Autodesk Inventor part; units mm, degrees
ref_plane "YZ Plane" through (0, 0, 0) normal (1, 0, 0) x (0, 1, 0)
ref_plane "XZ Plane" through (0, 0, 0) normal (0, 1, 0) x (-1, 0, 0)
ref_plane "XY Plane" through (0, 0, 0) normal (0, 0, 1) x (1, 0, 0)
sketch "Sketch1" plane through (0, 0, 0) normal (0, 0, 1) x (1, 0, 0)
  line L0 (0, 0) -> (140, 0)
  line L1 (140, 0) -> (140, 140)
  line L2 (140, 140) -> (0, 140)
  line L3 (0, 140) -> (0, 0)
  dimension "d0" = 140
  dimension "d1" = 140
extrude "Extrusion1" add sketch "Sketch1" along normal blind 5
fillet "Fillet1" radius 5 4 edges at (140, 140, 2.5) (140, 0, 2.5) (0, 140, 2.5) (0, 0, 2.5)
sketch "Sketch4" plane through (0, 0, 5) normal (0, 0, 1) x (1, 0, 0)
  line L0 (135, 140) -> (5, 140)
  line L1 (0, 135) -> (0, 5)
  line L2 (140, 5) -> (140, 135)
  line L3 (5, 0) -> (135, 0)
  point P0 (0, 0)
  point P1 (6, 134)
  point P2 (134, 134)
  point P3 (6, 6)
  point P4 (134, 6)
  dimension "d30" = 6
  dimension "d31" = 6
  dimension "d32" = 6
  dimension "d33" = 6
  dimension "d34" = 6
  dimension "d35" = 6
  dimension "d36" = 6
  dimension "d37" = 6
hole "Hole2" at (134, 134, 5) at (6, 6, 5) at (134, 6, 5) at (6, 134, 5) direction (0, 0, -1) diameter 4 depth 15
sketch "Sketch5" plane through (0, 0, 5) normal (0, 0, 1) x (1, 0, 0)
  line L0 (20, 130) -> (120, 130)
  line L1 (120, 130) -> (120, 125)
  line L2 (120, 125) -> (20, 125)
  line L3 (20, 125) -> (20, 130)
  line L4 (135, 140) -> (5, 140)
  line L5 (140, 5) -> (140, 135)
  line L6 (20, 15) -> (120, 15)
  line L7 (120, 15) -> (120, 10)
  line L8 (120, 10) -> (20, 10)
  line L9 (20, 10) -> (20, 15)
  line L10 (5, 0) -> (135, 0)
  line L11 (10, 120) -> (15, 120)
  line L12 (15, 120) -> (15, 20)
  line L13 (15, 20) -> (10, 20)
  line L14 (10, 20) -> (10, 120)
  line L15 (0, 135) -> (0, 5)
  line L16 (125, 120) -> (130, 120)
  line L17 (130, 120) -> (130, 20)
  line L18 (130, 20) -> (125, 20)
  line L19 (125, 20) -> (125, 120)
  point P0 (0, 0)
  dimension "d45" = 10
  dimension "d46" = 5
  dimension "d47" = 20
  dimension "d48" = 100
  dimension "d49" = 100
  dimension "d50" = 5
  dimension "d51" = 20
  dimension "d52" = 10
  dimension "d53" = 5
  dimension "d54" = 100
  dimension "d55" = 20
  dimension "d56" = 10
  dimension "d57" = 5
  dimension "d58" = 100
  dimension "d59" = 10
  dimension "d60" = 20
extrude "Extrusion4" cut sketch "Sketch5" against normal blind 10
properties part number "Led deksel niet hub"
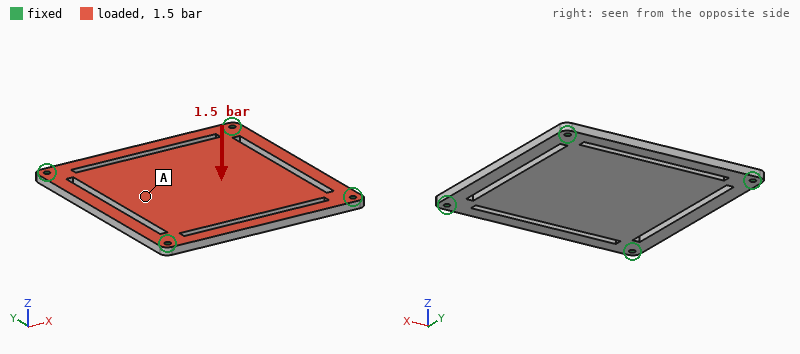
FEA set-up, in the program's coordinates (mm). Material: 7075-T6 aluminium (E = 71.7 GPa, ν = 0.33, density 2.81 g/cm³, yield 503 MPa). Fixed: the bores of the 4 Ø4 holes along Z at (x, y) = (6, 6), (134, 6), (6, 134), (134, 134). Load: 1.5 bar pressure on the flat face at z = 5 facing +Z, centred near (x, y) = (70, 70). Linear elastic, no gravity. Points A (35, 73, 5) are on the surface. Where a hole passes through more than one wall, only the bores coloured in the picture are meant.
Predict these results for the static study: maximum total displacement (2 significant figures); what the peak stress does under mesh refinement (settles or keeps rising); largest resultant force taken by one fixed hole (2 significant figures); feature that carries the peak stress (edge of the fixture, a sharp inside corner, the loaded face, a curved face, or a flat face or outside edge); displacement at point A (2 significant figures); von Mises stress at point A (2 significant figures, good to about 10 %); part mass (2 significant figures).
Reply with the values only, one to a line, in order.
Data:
0.52 mm
keeps rising
660 N
edge of the fixture
0.44 mm
37 MPa
250 g
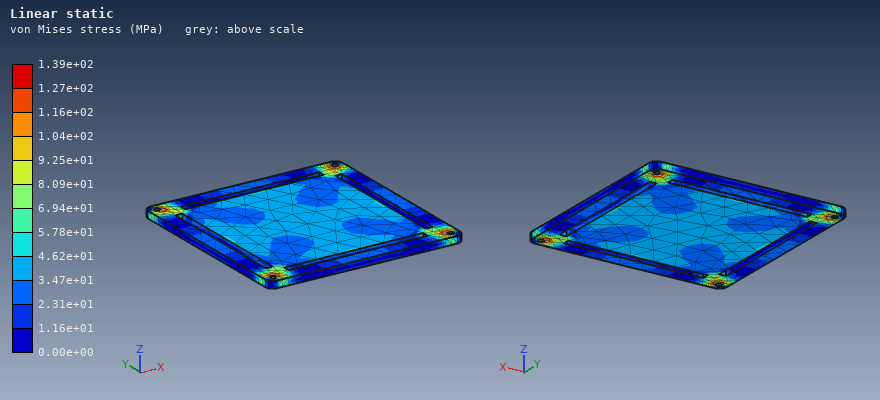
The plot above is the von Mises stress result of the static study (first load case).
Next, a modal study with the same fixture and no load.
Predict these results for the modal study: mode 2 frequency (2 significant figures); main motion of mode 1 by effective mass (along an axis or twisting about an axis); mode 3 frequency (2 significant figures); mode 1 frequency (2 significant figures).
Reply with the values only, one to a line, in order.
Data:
1600 Hz
along Z
1600 Hz
830 Hz
